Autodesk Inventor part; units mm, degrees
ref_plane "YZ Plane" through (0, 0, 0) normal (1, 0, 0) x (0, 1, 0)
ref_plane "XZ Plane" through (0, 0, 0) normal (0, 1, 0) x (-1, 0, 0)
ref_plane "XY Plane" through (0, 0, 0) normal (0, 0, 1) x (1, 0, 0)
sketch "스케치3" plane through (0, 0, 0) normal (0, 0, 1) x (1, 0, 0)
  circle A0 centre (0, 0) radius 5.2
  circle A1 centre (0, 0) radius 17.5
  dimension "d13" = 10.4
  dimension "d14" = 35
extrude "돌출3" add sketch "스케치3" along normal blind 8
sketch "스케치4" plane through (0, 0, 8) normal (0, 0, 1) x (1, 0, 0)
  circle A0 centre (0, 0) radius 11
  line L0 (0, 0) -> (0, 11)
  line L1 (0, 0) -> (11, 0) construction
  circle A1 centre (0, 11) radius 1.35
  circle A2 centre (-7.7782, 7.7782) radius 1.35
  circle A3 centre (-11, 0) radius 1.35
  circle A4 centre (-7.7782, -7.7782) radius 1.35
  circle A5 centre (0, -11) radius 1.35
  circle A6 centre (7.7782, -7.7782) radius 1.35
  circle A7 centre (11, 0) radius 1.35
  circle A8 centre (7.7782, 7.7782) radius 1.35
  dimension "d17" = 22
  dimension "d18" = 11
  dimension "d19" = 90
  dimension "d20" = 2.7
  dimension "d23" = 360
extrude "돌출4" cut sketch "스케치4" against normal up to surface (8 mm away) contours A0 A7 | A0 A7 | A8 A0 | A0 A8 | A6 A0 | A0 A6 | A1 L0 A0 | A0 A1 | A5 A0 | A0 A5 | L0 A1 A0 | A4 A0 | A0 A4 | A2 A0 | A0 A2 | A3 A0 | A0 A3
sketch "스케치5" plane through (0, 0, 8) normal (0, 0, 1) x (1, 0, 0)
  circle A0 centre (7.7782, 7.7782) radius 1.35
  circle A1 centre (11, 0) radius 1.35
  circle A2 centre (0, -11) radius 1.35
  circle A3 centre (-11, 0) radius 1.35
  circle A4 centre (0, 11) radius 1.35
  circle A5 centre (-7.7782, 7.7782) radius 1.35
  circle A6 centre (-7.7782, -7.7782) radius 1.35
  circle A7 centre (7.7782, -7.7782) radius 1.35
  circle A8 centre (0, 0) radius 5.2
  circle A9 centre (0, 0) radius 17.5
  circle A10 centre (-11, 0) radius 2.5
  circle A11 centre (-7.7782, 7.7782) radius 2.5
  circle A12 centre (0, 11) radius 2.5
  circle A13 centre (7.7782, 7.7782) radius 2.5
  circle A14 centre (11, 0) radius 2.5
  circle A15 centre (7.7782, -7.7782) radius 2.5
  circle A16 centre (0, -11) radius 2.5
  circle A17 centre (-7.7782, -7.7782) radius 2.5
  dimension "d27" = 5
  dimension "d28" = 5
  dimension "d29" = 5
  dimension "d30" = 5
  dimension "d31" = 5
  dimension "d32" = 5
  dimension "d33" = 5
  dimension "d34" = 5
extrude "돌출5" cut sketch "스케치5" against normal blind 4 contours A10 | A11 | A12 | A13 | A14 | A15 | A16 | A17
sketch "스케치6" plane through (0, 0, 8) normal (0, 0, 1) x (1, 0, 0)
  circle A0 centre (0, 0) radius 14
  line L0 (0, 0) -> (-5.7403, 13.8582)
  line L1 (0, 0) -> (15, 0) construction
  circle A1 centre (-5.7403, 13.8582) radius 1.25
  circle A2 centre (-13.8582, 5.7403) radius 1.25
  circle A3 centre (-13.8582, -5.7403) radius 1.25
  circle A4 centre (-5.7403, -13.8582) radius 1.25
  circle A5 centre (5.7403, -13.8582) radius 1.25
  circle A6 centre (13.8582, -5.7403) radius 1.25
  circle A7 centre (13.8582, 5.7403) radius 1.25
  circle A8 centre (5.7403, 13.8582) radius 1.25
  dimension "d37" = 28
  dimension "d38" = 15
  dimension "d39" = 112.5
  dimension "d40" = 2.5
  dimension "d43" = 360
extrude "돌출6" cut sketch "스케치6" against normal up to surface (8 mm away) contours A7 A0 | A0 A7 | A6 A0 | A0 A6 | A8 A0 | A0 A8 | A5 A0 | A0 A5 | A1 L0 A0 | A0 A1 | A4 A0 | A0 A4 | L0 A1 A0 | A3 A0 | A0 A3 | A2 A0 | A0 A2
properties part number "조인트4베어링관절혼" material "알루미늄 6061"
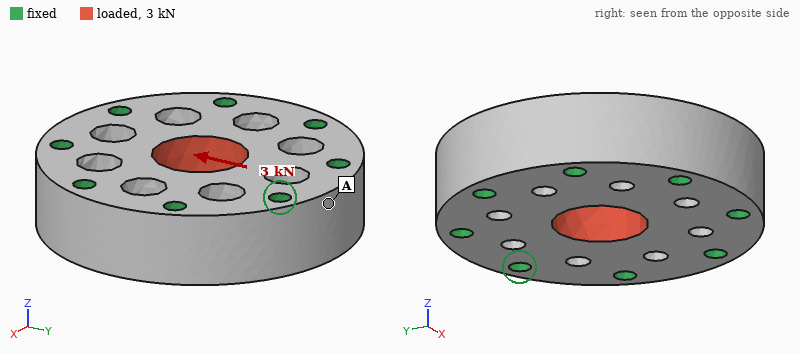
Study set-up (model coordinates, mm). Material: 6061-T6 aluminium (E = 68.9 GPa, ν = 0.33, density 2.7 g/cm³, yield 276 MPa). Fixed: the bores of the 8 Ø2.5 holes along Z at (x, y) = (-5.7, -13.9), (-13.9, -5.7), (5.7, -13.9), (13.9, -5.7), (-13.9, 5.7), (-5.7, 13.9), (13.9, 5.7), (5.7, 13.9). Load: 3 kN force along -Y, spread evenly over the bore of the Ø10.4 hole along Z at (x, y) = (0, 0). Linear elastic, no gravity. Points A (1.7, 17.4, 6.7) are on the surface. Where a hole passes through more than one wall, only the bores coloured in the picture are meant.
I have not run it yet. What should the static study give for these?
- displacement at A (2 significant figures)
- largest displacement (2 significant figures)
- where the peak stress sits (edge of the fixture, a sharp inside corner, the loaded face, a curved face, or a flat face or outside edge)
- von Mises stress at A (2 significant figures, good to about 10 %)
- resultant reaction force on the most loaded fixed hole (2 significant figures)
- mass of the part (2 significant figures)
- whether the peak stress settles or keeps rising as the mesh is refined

0.37 µm
2.2 µm
edge of the fixture
3.5 MPa
580 N
16 g
keeps rising
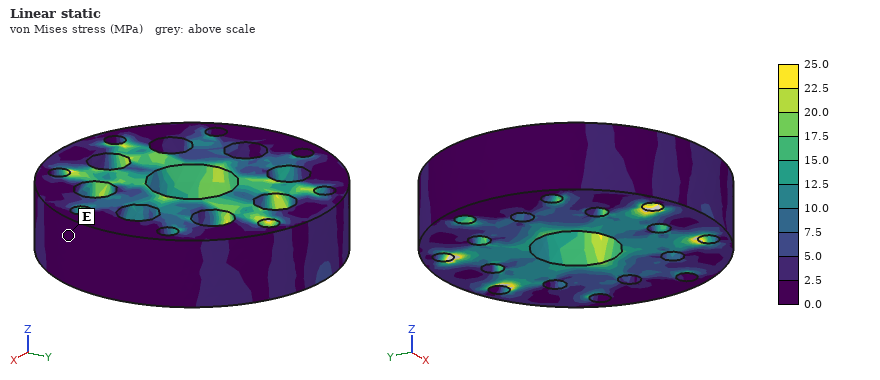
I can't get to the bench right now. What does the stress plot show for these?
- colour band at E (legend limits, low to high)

0.0 to 2.5 MPa
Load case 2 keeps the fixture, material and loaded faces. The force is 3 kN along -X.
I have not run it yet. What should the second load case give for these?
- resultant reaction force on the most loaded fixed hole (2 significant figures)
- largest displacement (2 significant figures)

580 N
2.2 µm
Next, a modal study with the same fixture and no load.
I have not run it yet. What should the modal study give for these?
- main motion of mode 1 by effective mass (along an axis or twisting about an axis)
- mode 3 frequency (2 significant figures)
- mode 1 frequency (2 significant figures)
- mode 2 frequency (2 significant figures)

along Z
77 kHz
58 kHz
77 kHz
